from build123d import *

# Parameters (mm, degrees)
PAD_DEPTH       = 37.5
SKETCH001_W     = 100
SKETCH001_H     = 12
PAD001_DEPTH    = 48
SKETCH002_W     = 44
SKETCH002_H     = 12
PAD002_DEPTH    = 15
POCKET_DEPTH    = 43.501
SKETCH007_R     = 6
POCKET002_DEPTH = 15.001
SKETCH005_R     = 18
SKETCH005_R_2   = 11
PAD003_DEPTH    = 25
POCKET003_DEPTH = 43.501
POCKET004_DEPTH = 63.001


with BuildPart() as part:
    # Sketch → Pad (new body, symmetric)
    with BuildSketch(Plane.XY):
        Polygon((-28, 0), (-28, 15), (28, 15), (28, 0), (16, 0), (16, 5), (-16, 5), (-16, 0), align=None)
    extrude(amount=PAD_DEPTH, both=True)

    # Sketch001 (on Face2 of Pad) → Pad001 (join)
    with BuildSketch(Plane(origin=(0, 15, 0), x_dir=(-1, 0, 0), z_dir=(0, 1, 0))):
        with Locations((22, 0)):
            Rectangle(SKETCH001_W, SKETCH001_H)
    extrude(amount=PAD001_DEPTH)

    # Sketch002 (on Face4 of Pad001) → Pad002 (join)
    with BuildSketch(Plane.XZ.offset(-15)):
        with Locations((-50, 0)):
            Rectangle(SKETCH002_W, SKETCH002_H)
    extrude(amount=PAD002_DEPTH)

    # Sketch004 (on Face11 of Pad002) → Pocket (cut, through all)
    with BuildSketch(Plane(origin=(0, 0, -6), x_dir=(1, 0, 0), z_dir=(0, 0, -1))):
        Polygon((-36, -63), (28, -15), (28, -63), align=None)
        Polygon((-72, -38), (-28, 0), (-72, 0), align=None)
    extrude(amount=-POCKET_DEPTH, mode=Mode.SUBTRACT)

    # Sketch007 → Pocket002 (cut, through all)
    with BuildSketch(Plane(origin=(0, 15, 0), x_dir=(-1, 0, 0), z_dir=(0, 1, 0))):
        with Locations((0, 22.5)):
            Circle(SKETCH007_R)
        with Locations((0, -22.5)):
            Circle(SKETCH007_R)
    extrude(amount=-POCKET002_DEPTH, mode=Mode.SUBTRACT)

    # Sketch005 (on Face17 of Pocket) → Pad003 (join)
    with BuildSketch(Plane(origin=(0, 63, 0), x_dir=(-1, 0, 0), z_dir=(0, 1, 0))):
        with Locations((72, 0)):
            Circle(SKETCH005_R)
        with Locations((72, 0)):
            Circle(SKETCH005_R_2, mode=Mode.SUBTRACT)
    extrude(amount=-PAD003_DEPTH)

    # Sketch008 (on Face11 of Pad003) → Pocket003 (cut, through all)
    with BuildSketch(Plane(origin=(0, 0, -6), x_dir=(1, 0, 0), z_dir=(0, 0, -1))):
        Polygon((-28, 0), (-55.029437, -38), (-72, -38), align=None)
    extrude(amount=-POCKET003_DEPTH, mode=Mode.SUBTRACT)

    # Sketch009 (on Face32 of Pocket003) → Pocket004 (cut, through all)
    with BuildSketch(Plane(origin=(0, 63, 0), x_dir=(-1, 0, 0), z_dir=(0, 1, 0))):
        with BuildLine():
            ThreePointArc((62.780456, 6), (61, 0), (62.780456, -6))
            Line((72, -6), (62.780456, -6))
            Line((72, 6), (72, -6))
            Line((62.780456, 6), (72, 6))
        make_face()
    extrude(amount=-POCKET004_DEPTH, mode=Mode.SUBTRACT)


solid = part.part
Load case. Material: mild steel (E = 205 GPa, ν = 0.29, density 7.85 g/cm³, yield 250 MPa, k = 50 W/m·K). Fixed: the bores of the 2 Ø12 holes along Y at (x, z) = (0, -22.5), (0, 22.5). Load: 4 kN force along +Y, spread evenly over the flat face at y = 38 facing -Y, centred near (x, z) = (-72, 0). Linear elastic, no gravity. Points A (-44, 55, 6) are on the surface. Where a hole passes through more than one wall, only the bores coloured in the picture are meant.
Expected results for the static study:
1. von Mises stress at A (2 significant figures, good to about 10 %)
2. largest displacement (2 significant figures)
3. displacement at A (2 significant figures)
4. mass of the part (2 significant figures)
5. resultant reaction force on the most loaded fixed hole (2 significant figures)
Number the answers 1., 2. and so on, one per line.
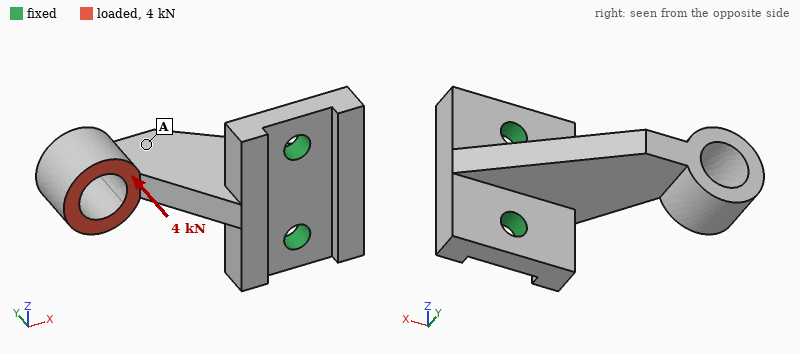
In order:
1. 30 MPa
2. 0.22 mm
3. 0.10 mm
4. 730 g
5. 2.6 kN
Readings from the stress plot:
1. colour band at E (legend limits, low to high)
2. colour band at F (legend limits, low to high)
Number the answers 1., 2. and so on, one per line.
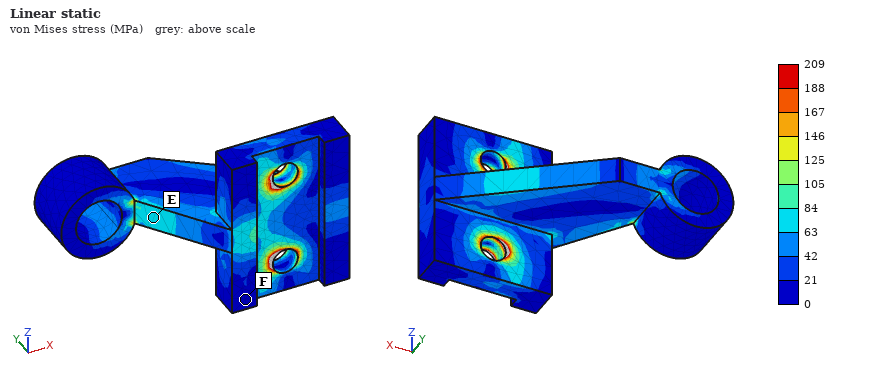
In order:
1. 63 to 84 MPa
2. 0 to 21 MPa
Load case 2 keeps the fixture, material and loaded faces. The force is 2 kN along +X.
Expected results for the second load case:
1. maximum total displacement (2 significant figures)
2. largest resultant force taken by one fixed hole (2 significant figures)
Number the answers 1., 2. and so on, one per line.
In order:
1. 25 µm
2. 1.0 kN
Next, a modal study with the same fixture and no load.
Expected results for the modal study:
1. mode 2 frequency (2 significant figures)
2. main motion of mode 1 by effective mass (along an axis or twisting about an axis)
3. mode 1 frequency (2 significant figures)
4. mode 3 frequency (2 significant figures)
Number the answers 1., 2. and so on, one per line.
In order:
1. 1800 Hz
2. along Z
3. 1200 Hz
4. 3700 Hz
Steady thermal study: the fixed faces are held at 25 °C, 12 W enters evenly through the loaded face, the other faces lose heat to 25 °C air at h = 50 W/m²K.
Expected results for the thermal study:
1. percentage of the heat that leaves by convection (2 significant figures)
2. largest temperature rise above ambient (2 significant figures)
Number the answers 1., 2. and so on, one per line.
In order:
1. 66 %
2. 27 K
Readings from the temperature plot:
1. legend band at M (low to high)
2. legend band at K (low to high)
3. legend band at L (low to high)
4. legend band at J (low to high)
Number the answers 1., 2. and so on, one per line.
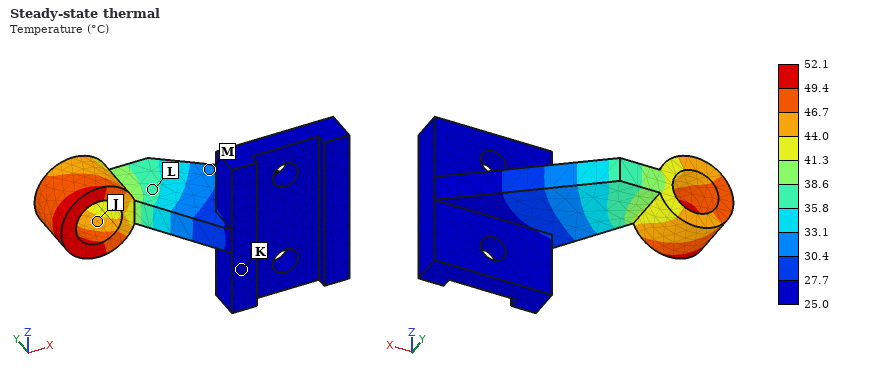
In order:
1. 30.4 to 33.1 °C
2. 25.0 to 27.7 °C
3. 35.8 to 38.6 °C
4. 44.0 to 46.7 °C
